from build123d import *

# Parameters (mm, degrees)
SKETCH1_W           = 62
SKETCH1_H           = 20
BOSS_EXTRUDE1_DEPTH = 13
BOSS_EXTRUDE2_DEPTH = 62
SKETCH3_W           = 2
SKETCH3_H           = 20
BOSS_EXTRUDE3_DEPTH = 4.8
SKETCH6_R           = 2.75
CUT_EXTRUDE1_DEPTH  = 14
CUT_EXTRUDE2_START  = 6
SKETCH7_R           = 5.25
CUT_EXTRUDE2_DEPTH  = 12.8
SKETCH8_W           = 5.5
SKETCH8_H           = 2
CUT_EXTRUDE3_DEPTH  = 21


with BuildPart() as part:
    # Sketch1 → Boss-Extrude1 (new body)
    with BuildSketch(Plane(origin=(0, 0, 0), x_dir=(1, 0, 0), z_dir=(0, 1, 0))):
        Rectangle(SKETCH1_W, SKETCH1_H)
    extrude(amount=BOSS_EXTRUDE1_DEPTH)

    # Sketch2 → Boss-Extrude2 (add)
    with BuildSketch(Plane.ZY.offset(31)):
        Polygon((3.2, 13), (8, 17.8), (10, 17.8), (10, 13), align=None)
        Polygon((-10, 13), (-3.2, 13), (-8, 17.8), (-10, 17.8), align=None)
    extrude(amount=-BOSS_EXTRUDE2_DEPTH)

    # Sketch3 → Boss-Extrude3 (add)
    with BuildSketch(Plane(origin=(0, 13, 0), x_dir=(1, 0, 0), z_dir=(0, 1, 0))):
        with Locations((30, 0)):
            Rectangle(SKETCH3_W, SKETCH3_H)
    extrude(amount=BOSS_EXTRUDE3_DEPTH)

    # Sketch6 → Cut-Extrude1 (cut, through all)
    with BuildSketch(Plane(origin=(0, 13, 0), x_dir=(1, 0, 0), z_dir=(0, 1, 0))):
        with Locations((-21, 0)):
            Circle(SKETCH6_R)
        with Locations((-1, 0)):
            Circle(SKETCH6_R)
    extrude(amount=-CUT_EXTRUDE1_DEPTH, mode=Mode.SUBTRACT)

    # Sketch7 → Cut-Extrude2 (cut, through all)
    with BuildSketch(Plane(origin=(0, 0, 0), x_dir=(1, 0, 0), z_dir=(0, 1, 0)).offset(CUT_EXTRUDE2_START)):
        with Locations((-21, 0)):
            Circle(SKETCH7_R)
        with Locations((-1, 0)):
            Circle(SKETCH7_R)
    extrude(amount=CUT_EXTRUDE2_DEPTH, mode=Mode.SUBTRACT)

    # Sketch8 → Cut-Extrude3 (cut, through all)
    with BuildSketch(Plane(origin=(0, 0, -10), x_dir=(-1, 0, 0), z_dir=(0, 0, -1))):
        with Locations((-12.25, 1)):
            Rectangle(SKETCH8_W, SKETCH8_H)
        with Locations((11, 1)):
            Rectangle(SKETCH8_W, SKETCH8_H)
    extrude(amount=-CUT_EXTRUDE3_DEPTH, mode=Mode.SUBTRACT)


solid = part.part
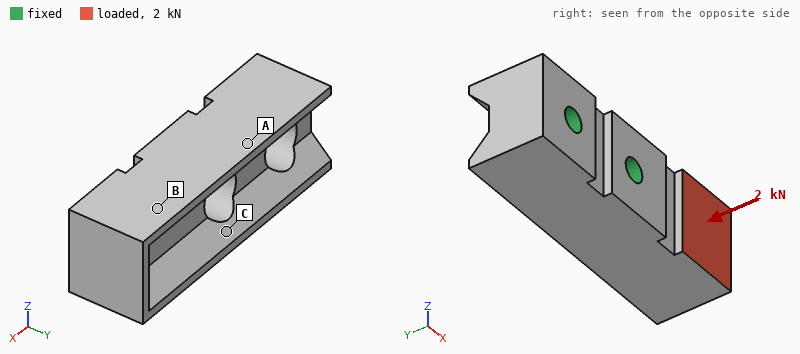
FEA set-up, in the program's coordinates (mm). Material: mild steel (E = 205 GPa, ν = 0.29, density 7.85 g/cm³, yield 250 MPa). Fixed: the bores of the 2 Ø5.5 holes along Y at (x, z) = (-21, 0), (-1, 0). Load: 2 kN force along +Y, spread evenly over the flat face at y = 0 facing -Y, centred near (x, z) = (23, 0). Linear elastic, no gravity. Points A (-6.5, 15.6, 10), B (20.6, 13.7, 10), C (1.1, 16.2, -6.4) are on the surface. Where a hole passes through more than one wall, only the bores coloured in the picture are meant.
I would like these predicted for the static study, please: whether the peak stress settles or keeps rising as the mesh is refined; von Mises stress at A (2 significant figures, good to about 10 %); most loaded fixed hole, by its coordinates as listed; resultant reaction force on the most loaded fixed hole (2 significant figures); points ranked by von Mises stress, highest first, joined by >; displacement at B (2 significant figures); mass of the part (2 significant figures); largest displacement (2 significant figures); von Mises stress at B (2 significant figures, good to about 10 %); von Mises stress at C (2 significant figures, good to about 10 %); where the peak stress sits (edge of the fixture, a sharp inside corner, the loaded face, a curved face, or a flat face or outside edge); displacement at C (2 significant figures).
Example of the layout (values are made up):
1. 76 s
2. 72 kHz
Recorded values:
1. keeps rising
2. 37 MPa
3. (-1, 0)
4. 3.9 kN
5. C > A > B
6. 18 µm
7. 130 g
8. 28 µm
9. 14 MPa
10. 60 MPa
11. edge of the fixture
12. 5.8 µm
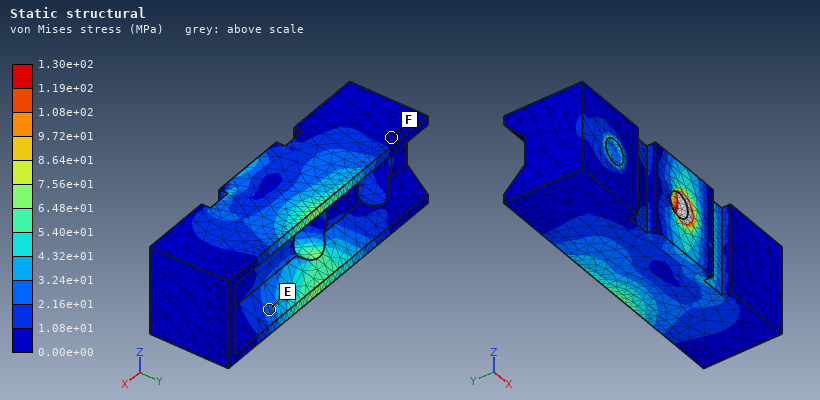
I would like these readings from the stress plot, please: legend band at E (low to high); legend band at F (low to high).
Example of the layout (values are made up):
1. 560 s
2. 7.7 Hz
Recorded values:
1. 2.16e+01 to 3.24e+01 MPa
2. 0.00e+00 to 1.08e+01 MPa
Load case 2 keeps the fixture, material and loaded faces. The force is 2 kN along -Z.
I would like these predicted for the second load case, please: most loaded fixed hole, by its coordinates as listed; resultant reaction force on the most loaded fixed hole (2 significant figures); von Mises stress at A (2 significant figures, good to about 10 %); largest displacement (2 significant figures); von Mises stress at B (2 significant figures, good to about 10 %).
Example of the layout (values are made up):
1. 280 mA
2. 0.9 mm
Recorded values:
1. (-1, 0)
2. 3.6 kN
3. 24 MPa
4. 24 µm
5. 12 MPa
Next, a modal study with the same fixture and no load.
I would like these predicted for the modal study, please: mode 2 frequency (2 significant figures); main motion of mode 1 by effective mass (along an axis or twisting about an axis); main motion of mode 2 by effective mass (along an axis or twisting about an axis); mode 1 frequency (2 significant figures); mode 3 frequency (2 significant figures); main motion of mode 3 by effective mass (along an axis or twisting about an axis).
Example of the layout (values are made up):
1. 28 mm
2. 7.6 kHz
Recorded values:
1. 8000 Hz
2. along Y
3. along Z
4. 7400 Hz
5. 12 kHz
6. twisting about X
